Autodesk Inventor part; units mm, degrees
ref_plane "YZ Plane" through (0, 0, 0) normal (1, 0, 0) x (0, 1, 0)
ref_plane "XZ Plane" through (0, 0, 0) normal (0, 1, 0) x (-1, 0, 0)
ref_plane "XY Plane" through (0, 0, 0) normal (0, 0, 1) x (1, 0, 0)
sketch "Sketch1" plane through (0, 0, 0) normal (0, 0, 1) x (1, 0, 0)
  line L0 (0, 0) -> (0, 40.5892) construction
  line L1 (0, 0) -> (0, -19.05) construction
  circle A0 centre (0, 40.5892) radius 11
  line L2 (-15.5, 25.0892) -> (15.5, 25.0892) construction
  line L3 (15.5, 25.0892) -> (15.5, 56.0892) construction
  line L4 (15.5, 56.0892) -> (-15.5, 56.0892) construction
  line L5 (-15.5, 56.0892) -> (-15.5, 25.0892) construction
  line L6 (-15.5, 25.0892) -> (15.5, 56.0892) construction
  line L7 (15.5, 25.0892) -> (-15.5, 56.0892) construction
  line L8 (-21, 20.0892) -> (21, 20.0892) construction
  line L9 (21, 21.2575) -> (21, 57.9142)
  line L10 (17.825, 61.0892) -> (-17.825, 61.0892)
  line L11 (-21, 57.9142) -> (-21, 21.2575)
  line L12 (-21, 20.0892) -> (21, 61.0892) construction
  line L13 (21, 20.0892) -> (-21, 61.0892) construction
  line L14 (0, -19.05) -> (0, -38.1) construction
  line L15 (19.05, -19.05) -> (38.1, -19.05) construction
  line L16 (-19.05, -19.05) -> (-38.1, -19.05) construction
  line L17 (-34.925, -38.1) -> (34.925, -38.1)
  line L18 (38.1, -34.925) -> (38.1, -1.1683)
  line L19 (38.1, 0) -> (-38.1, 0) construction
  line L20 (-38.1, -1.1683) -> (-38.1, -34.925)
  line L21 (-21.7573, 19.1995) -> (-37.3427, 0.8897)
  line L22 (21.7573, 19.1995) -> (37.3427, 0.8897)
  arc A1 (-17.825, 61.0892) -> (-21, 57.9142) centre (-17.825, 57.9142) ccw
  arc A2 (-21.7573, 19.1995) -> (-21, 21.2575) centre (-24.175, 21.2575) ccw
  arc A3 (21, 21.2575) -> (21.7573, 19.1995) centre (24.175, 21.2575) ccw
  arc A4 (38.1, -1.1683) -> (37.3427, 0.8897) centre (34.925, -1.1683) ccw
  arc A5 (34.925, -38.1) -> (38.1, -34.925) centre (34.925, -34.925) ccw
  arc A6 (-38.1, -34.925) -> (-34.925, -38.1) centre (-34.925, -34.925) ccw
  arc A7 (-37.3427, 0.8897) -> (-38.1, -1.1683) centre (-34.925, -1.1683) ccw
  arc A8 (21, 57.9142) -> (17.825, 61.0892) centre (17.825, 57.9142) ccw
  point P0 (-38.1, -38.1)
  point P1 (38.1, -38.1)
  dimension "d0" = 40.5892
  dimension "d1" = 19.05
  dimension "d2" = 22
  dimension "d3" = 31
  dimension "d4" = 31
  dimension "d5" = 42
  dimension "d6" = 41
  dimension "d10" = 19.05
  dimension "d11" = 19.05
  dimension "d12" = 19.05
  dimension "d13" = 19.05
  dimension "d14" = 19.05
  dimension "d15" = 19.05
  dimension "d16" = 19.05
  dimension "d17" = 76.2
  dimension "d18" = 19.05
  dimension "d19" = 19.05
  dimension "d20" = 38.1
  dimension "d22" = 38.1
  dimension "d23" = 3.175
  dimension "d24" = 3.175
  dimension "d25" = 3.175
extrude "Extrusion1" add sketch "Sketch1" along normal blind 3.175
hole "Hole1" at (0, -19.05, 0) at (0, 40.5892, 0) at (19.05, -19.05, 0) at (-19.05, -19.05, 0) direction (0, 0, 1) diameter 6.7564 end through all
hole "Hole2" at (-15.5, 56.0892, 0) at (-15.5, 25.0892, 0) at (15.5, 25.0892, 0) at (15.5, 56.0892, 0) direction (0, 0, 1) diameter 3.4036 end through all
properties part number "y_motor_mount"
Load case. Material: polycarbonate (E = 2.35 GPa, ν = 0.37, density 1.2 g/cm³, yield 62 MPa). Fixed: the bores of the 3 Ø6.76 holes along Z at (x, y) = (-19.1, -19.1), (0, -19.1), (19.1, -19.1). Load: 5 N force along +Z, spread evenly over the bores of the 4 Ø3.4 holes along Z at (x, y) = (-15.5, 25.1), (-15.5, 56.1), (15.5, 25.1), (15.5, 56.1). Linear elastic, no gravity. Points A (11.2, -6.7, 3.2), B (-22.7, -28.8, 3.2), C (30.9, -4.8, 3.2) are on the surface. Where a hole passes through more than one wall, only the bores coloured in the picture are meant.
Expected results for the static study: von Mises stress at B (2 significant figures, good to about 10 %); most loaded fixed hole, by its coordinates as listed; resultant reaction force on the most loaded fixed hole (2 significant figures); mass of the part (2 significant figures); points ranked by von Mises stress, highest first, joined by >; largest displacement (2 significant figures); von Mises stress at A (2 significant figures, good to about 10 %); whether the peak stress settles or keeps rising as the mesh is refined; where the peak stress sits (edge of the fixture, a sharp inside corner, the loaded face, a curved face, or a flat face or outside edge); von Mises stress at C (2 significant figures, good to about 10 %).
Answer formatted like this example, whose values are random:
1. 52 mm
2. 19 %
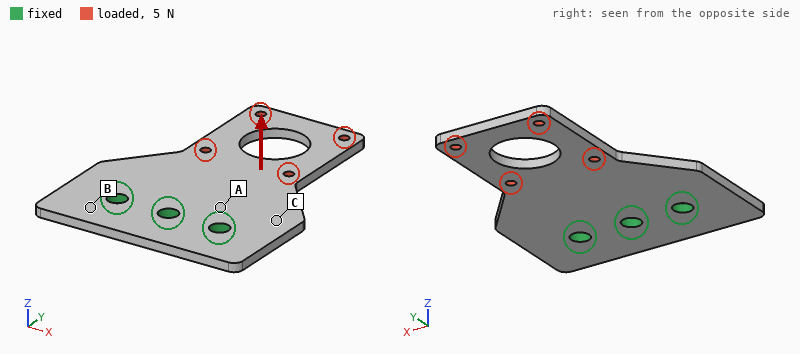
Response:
1. 0.33 MPa
2. (0, -19.1)
3. 3.0 N
4. 20 g
5. A > C > B
6. 1.4 mm
7. 1.9 MPa
8. keeps rising
9. edge of the fixture
10. 1.4 MPa
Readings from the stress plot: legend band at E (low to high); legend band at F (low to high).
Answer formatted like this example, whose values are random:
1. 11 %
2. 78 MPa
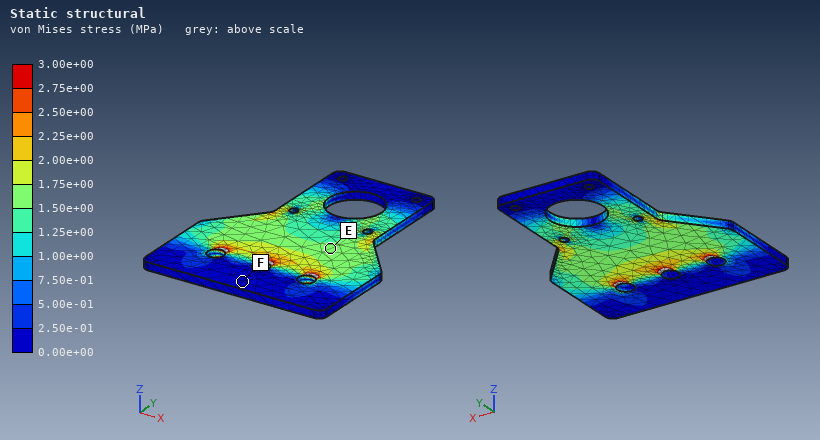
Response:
1. 1.50e+00 to 1.75e+00 MPa
2. 0.00e+00 to 2.50e-01 MPa
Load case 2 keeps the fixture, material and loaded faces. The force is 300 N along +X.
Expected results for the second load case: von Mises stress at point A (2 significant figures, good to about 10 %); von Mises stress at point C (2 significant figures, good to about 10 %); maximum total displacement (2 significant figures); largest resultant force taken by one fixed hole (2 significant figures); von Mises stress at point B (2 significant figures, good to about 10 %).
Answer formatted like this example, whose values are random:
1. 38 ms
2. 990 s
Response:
1. 4.8 MPa
2. 3.0 MPa
3. 0.65 mm
4. 430 N
5. 2.3 MPa
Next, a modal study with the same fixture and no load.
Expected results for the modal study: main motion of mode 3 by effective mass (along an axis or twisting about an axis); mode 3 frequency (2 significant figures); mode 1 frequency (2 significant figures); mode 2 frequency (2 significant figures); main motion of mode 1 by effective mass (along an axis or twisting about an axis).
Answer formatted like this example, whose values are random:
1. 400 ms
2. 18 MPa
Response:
1. along Z
2. 700 Hz
3. 160 Hz
4. 510 Hz
5. along Z
